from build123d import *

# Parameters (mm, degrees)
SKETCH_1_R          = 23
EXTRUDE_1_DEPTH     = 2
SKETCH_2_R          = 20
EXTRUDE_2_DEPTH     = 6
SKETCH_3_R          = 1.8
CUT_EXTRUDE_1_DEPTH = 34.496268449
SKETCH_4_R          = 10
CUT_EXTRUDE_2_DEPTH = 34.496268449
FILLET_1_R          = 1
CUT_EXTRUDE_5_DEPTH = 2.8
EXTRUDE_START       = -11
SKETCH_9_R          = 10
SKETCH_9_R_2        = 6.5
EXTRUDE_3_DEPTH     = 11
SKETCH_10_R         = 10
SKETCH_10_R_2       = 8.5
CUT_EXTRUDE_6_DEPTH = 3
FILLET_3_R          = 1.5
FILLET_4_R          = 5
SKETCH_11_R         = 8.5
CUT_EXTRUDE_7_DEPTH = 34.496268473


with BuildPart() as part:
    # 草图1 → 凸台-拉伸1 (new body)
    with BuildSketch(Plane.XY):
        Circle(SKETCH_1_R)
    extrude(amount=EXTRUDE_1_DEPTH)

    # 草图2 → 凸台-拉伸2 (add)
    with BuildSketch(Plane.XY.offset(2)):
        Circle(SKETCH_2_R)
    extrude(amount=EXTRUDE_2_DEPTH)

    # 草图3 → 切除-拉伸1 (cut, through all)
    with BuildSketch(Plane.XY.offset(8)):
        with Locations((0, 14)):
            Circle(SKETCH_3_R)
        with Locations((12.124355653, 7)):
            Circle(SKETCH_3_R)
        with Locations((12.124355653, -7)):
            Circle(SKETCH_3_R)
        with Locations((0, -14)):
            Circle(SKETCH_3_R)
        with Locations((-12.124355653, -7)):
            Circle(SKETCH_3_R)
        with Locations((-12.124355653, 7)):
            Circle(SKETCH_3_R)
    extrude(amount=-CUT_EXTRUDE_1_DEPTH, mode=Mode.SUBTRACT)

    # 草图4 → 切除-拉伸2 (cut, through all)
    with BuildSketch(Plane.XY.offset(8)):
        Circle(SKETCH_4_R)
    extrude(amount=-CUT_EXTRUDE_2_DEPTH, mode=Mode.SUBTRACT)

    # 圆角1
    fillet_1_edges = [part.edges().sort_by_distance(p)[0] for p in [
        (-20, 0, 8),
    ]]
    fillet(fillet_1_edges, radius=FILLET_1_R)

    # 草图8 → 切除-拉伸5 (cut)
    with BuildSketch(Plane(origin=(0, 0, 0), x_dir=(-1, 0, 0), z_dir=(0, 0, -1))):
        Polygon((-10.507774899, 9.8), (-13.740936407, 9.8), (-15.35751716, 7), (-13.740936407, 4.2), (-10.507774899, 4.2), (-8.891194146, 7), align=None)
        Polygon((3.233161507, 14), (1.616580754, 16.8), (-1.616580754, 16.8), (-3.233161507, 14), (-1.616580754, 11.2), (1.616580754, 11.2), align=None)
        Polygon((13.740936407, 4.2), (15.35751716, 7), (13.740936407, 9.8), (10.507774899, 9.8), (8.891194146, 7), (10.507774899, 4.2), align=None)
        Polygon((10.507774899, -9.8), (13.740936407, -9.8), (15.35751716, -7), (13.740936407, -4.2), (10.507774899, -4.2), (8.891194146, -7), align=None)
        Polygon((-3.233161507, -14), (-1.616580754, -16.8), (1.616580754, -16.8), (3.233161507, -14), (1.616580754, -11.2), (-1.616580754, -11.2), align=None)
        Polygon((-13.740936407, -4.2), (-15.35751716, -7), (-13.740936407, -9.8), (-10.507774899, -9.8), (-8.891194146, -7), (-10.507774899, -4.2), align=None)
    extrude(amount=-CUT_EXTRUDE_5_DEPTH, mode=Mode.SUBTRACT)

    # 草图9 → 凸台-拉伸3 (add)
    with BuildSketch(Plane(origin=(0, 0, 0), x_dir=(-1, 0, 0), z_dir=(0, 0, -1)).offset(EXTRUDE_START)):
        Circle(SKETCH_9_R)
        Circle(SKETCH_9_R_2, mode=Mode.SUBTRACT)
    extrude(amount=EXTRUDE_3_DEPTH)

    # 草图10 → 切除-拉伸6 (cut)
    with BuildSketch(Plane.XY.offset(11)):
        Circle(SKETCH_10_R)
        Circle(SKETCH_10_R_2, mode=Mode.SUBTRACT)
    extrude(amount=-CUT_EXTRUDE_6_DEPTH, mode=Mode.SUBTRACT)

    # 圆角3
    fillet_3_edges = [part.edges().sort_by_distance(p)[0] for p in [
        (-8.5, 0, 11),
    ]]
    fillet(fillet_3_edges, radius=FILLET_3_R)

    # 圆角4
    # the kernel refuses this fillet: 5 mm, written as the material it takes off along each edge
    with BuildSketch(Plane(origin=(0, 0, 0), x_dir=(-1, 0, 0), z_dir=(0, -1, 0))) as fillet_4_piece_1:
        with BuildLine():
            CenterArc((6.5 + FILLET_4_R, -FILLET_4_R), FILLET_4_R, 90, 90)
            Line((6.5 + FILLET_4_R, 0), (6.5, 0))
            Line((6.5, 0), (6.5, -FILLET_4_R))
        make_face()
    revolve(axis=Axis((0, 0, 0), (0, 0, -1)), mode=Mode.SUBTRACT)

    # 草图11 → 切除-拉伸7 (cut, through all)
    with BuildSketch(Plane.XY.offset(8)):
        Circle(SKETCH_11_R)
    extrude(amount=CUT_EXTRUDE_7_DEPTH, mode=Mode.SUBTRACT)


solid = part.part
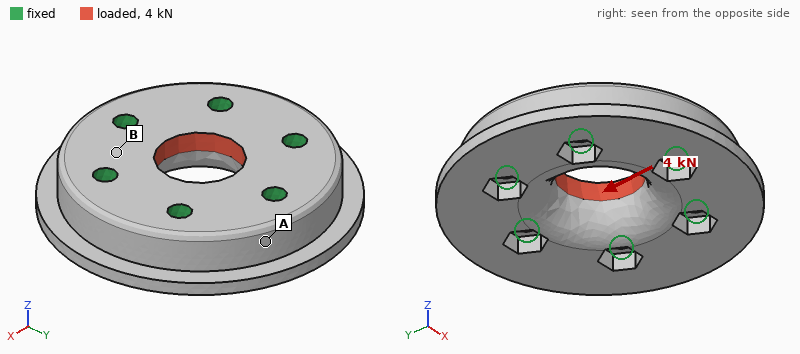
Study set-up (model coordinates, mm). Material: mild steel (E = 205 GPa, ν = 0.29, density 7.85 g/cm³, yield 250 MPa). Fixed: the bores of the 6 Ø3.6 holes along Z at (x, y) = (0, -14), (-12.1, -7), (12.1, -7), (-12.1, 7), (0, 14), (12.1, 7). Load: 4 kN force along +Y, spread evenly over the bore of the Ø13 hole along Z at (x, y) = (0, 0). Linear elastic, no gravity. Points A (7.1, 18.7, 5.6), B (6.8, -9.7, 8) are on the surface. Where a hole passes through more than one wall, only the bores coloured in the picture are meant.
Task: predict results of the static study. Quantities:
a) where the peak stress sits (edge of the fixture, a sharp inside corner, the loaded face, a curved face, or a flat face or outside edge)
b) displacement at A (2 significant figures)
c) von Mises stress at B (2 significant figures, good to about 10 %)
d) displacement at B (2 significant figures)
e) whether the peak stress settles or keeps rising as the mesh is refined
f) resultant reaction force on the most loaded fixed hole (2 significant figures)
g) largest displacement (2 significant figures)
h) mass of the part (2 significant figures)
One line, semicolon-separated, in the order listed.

a sharp inside corner; 0.19 µm; 12 MPa; 0.40 µm; keeps rising; 950 N; 1.2 µm; 69 g
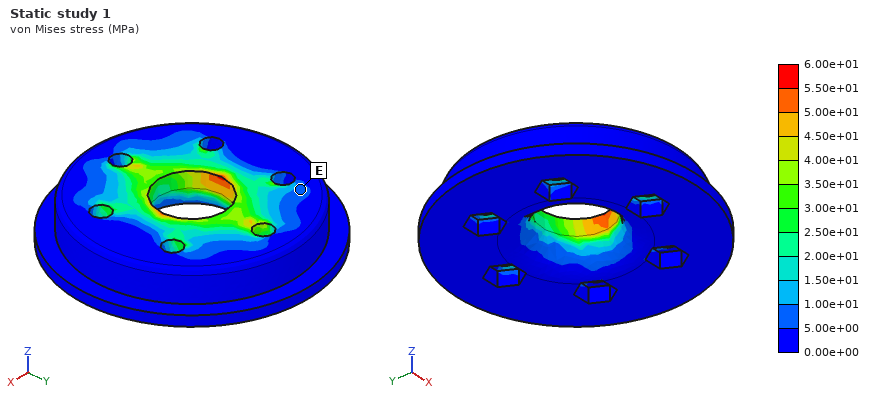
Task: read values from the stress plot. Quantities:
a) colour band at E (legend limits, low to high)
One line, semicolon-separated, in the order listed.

5.00e+00 to 1.00e+01 MPa
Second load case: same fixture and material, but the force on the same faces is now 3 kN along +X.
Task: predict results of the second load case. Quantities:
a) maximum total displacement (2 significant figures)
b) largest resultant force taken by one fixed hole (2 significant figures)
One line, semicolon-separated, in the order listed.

0.93 µm; 640 N
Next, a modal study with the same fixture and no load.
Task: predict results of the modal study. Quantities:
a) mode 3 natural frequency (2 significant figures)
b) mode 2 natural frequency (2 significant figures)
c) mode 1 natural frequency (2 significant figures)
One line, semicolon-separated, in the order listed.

46 kHz; 45 kHz; 45 kHz
